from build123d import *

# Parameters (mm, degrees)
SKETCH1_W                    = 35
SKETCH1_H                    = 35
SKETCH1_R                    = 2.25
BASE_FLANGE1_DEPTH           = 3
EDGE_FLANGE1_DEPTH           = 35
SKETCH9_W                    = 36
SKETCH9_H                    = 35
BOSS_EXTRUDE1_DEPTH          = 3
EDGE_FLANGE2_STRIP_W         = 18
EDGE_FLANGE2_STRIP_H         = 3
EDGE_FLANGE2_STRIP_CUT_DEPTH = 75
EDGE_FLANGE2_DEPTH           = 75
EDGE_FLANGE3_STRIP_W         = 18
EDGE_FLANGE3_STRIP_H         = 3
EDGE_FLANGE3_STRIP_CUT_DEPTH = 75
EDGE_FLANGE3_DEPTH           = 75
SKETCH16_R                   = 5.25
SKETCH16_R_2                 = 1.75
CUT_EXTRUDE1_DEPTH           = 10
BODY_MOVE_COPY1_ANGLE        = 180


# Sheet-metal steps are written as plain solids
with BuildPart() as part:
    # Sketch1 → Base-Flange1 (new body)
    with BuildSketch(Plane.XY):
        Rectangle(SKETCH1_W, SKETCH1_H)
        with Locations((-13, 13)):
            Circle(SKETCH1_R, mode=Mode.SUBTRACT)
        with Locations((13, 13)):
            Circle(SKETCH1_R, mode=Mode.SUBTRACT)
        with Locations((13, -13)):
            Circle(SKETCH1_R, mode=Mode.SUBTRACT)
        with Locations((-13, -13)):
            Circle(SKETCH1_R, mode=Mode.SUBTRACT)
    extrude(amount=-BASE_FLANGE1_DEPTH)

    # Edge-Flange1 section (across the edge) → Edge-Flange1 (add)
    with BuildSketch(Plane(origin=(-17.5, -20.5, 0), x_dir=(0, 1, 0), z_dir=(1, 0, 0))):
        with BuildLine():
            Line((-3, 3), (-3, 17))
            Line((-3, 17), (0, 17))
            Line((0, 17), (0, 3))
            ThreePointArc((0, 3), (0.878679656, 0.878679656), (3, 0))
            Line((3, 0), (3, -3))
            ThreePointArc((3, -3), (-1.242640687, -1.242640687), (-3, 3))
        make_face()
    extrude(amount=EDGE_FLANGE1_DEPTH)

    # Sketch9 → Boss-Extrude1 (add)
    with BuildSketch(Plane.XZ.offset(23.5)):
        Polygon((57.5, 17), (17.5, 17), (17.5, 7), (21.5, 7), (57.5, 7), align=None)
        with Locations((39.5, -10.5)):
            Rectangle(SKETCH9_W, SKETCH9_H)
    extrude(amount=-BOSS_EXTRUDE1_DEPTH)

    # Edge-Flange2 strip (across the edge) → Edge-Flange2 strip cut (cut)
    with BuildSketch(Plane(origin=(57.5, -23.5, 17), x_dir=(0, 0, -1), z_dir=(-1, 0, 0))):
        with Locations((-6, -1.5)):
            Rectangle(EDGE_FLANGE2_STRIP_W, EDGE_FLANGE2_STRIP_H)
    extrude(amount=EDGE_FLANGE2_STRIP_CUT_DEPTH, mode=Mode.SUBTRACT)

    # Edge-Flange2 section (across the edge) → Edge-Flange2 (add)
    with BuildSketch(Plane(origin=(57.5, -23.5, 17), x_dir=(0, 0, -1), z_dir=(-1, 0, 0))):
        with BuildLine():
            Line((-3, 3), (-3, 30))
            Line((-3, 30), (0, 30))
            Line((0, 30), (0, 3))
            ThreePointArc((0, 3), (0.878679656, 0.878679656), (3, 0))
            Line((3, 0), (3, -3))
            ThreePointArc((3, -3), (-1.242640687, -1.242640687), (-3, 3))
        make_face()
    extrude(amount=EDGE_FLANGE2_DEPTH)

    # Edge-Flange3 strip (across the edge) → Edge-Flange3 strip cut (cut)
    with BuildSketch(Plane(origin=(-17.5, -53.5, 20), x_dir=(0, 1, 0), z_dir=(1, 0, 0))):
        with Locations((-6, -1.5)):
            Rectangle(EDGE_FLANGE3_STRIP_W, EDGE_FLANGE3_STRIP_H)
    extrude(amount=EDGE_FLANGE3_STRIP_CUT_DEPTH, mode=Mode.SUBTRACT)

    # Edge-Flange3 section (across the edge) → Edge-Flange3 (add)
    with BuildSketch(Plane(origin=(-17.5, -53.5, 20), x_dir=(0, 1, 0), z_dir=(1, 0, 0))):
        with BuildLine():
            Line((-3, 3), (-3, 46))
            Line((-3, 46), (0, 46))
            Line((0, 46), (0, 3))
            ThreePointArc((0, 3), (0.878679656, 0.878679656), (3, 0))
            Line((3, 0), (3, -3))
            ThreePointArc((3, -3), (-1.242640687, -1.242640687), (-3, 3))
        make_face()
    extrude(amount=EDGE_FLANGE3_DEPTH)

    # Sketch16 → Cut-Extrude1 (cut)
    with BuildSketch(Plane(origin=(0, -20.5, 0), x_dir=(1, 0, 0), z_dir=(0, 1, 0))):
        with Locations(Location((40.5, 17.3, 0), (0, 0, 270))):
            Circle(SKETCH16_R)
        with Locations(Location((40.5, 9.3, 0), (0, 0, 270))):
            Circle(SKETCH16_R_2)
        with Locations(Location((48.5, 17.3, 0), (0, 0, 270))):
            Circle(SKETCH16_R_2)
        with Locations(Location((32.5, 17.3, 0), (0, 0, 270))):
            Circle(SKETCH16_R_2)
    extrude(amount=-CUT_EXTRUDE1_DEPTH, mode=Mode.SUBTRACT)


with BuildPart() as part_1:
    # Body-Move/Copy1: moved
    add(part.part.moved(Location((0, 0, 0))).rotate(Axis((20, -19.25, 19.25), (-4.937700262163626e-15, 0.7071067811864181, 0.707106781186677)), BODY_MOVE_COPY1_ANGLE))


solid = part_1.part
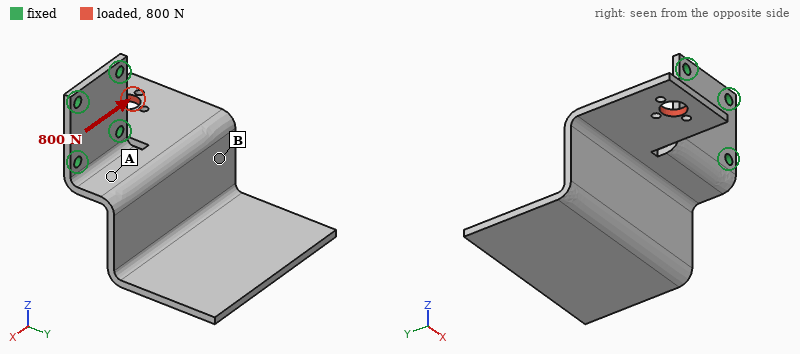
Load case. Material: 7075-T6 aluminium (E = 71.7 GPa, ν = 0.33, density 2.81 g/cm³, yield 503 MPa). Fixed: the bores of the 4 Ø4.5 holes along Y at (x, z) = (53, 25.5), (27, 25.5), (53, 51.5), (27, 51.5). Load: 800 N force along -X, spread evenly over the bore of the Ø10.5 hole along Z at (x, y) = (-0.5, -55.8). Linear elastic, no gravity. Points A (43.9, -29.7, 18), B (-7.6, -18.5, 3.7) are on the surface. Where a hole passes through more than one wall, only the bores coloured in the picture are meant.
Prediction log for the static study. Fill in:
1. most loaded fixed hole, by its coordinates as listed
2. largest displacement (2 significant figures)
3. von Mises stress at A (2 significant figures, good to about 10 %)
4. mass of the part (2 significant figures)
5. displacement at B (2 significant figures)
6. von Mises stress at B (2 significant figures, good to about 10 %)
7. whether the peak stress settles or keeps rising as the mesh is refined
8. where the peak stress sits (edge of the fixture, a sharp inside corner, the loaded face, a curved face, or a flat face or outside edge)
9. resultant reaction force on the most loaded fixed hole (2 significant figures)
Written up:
(27, 25.5)
0.74 mm
50 MPa
78 g
0.43 mm
20 MPa
keeps rising
a sharp inside corner
740 N
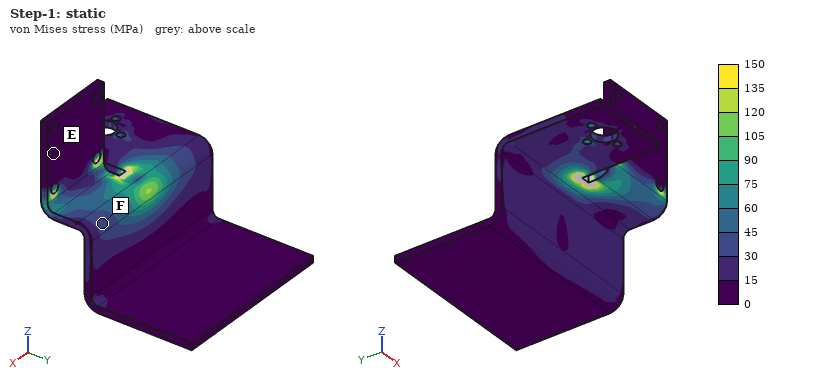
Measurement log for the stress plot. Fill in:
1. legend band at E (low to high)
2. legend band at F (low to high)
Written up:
0 to 15 MPa
30 to 45 MPa
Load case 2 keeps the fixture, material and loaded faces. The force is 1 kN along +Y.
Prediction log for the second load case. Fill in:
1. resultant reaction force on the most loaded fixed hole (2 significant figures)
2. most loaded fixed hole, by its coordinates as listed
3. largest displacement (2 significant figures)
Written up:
2.1 kN
(27, 25.5)
1.4 mm
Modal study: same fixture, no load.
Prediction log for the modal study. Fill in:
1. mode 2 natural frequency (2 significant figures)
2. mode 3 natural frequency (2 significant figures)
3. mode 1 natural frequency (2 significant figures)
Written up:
570 Hz
700 Hz
220 Hz
